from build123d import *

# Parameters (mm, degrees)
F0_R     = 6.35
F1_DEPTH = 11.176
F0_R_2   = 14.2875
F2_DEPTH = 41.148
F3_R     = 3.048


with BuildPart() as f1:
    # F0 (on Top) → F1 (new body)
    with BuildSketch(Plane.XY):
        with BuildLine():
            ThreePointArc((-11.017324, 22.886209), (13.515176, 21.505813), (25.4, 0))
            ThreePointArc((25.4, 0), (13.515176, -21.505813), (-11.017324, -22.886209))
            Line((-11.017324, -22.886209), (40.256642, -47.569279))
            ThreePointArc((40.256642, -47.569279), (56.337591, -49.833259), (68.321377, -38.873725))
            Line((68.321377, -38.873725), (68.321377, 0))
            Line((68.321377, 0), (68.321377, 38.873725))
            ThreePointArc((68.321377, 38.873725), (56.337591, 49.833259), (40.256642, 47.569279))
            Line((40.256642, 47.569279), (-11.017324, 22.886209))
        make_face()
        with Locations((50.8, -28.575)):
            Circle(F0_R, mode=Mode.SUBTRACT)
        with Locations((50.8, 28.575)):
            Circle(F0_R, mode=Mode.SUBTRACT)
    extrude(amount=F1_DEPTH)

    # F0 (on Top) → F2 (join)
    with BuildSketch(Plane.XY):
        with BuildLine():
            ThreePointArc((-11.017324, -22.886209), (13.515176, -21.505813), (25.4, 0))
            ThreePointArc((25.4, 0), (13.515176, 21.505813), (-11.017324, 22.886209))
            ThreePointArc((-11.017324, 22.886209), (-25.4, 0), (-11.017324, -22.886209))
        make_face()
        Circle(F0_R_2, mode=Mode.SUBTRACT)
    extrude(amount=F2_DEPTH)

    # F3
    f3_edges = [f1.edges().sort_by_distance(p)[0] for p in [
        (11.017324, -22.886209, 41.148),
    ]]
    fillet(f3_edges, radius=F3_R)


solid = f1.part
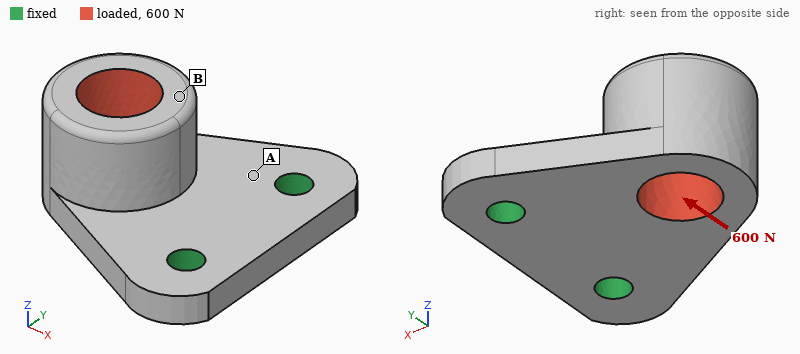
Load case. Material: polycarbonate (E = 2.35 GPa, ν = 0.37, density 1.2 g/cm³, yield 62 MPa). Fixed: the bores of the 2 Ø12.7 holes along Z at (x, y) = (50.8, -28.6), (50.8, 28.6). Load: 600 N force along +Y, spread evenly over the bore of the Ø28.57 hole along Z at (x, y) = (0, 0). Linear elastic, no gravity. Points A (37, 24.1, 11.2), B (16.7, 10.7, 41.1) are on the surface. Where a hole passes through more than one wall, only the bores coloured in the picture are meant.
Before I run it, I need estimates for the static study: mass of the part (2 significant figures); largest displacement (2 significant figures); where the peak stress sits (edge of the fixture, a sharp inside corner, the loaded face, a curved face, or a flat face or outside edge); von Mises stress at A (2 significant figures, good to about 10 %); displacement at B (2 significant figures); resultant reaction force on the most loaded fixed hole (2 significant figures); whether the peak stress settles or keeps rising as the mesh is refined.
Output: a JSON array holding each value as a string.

["130 g", "0.23 mm", "edge of the fixture", "2.1 MPa", "0.18 mm", "570 N", "keeps rising"]
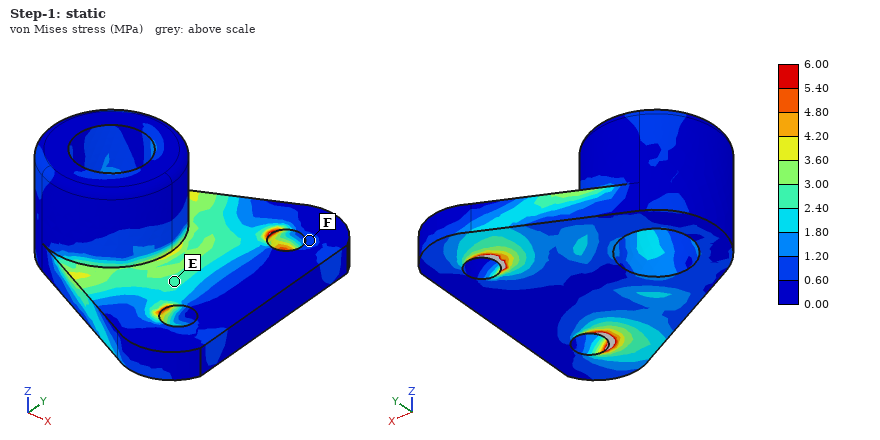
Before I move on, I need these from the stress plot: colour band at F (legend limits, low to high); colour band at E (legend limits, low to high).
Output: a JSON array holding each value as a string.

["0.60 to 1.20 MPa", "2.40 to 3.00 MPa"]
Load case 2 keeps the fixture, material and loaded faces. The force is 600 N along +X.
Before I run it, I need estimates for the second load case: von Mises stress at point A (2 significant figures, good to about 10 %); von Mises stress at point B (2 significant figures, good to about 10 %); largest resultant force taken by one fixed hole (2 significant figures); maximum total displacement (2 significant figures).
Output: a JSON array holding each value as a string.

["6.0 MPa", "0.77 MPa", "320 N", "0.89 mm"]
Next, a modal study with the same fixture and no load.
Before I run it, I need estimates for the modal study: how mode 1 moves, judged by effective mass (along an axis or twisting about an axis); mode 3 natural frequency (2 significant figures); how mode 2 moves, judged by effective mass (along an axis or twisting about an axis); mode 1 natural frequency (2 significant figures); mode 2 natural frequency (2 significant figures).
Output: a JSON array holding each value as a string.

["along Z", "1800 Hz", "along Y", "380 Hz", "1100 Hz"]
